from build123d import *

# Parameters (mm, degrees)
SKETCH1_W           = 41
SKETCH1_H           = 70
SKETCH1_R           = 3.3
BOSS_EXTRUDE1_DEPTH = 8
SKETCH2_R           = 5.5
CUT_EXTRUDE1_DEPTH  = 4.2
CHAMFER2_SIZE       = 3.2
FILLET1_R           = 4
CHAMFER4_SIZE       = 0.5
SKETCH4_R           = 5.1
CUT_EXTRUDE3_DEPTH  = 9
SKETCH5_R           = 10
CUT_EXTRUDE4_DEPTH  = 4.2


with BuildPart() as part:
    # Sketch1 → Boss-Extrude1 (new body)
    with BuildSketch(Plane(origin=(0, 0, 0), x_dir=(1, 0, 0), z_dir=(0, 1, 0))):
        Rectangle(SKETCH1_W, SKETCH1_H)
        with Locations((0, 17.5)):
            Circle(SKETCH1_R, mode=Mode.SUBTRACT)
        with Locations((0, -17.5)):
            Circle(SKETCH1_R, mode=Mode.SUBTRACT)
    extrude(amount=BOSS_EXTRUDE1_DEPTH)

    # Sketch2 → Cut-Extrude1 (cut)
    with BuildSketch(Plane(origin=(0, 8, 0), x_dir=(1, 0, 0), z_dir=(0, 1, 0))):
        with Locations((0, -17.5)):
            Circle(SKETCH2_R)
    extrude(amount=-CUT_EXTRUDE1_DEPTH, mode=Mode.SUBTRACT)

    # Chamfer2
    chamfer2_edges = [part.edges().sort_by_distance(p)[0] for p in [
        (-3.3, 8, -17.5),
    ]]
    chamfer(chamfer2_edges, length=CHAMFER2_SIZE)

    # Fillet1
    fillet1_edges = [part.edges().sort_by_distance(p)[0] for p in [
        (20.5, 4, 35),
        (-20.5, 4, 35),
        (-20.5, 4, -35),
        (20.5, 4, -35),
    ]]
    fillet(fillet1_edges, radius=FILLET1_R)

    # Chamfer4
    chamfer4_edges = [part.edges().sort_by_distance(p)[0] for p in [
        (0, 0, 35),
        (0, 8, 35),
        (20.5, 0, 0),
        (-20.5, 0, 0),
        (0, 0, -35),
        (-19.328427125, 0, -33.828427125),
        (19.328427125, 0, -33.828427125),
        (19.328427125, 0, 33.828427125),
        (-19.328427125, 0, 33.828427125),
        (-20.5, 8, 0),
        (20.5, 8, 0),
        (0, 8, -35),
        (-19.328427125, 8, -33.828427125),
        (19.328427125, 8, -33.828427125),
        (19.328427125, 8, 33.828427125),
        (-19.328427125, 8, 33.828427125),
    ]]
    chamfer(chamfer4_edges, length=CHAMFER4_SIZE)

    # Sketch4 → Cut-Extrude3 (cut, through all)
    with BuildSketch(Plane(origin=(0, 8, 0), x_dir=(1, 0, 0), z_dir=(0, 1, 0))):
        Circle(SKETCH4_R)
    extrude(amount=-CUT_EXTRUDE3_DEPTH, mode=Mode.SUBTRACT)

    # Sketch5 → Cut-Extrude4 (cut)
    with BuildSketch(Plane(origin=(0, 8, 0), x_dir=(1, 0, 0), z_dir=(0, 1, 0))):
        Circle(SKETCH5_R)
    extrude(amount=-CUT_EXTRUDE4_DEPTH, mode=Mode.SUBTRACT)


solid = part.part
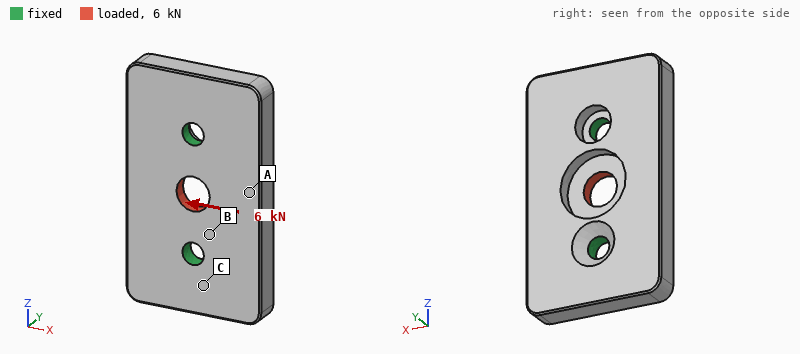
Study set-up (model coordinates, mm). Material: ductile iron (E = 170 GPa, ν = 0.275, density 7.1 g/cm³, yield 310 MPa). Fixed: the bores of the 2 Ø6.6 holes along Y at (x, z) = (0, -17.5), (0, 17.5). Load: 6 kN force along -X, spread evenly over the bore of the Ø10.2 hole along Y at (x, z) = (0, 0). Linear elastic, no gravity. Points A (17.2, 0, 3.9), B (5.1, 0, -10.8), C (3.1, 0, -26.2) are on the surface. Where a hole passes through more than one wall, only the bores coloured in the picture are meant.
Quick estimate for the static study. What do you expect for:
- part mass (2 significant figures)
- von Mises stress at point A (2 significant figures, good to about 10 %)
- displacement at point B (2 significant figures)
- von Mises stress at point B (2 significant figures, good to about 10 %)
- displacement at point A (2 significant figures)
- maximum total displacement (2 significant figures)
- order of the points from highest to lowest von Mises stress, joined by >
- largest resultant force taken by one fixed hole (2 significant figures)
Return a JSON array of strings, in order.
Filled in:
["140 g", "20 MPa", "2.0 µm", "33 MPa", "3.8 µm", "5.8 µm", "B > A > C", "3.0 kN"]
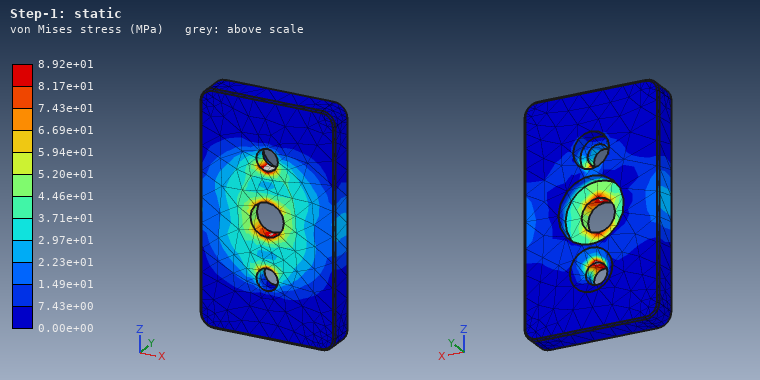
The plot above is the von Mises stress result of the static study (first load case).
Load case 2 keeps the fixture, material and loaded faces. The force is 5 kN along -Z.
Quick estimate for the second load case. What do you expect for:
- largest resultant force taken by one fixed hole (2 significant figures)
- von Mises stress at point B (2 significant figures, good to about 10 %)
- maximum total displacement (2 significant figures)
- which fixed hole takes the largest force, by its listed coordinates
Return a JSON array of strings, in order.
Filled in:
["2.6 kN", "27 MPa", "3.1 µm", "(0, -17.5)"]
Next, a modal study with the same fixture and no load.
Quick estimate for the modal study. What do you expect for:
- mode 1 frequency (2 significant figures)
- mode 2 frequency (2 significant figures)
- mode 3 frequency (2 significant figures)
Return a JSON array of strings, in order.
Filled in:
["6600 Hz", "9800 Hz", "10 kHz"]
